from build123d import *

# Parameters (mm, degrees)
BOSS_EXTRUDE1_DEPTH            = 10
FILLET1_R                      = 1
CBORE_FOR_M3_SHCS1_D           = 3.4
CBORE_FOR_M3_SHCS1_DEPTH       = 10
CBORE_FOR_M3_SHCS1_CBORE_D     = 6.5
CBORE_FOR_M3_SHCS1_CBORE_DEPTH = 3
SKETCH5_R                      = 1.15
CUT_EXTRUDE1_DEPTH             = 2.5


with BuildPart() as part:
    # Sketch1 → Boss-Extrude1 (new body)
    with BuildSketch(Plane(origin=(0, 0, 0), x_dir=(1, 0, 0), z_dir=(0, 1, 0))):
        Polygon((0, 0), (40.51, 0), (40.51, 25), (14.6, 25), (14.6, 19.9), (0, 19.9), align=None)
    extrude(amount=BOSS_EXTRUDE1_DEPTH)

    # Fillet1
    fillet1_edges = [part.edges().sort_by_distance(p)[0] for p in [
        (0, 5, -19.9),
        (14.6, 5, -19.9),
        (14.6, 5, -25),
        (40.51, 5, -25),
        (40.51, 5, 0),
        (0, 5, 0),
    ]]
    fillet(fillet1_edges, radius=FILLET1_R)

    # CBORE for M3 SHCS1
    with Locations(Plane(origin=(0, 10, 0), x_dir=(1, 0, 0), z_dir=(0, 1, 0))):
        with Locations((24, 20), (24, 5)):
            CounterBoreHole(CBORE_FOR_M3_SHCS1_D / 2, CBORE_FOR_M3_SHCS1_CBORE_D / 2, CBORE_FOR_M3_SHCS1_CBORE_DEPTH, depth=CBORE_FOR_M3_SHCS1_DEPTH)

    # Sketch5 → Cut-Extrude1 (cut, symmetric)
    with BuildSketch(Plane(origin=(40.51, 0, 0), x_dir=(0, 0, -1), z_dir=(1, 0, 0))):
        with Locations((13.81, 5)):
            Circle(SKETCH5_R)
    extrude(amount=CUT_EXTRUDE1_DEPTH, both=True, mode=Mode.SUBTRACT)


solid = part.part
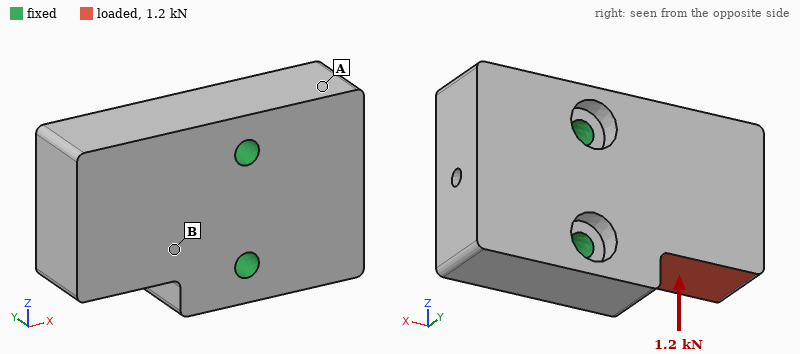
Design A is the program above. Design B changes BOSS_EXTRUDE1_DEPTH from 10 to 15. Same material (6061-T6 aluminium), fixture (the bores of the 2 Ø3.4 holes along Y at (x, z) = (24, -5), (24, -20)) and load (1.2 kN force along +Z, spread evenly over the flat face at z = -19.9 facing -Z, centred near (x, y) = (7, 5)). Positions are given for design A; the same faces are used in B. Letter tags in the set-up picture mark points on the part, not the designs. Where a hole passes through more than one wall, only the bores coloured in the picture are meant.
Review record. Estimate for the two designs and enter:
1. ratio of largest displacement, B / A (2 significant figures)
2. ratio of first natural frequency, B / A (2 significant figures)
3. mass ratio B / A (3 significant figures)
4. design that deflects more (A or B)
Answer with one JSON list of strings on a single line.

["0.85", "0.85", "1.48", "A"]
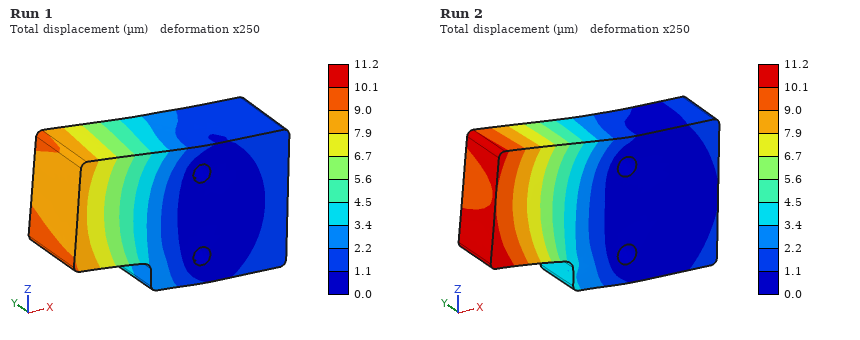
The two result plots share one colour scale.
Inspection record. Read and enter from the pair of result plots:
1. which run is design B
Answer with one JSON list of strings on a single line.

["Run 1"]
